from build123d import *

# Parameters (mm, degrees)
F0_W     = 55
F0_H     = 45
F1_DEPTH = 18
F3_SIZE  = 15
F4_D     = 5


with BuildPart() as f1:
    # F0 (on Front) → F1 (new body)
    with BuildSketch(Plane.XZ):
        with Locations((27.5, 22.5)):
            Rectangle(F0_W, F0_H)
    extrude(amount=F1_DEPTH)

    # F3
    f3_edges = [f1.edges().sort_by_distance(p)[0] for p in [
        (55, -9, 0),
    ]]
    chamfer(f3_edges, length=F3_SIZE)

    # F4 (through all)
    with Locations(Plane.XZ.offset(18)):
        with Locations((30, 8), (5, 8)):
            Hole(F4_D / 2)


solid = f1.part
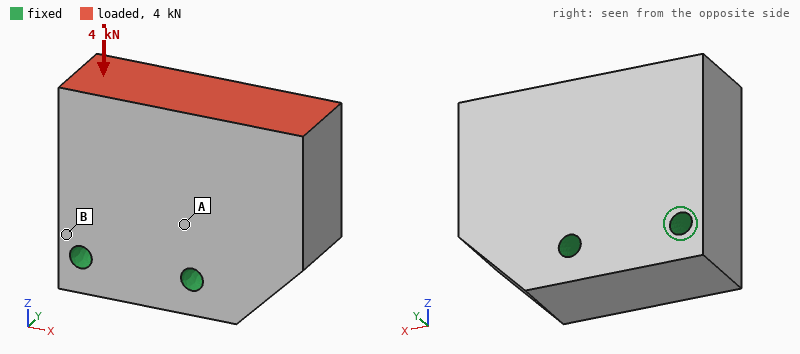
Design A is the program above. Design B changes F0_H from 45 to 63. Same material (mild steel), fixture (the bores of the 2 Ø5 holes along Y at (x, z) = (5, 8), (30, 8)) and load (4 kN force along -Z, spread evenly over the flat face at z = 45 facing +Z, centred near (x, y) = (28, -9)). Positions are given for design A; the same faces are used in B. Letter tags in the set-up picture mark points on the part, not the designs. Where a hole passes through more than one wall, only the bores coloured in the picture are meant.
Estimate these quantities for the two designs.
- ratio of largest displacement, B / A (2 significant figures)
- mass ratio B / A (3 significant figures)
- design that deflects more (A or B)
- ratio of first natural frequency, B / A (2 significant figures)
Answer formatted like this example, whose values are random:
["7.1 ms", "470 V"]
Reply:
["0.92", "1.43", "A", "0.73"]
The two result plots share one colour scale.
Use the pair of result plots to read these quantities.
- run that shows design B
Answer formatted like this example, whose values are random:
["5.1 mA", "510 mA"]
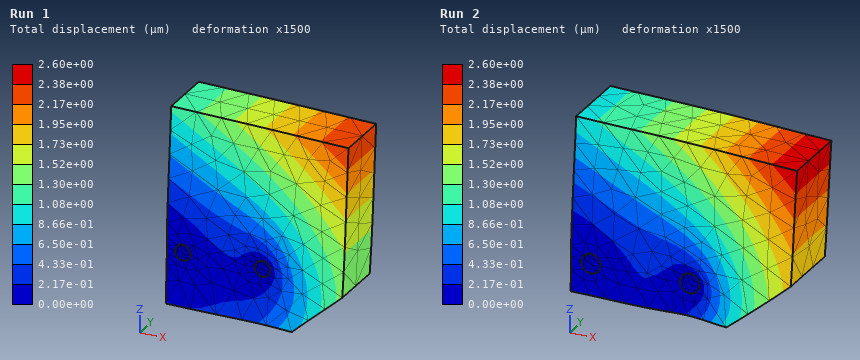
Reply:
["Run 1"]
